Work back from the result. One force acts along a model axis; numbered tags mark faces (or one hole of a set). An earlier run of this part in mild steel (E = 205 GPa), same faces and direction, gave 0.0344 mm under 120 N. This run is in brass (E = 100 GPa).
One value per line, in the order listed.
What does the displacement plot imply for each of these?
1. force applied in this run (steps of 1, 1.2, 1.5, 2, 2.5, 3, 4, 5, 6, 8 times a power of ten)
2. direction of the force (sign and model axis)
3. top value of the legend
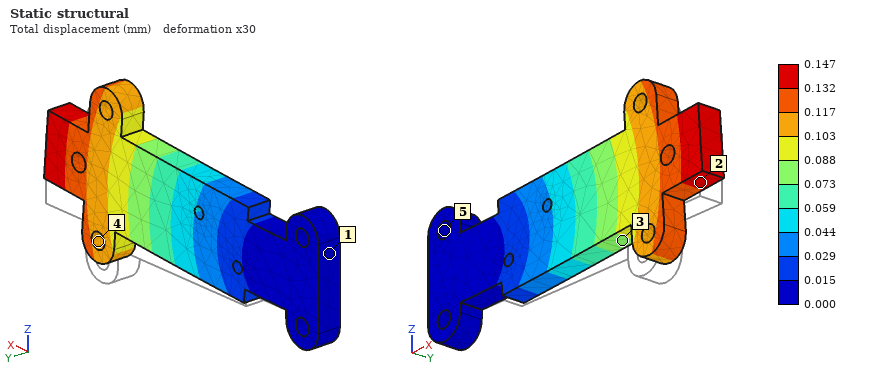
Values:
250 N
+Z
0.147 mm
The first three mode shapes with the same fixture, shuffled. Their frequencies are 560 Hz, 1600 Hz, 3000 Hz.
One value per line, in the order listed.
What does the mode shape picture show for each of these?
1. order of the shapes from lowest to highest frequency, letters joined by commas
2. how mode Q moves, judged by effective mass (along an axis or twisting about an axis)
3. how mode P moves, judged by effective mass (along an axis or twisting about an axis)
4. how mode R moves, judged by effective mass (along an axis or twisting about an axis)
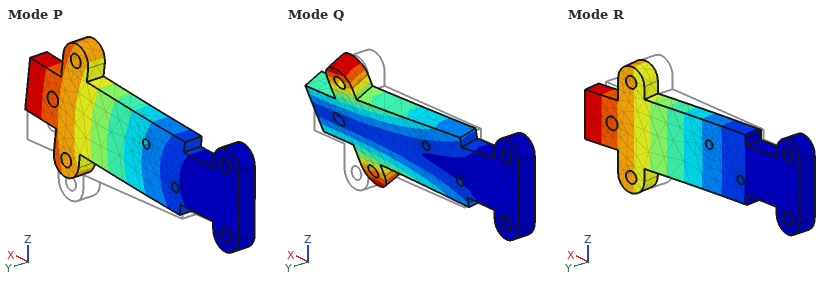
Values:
R, P, Q
twisting about X
along Z
along Y
